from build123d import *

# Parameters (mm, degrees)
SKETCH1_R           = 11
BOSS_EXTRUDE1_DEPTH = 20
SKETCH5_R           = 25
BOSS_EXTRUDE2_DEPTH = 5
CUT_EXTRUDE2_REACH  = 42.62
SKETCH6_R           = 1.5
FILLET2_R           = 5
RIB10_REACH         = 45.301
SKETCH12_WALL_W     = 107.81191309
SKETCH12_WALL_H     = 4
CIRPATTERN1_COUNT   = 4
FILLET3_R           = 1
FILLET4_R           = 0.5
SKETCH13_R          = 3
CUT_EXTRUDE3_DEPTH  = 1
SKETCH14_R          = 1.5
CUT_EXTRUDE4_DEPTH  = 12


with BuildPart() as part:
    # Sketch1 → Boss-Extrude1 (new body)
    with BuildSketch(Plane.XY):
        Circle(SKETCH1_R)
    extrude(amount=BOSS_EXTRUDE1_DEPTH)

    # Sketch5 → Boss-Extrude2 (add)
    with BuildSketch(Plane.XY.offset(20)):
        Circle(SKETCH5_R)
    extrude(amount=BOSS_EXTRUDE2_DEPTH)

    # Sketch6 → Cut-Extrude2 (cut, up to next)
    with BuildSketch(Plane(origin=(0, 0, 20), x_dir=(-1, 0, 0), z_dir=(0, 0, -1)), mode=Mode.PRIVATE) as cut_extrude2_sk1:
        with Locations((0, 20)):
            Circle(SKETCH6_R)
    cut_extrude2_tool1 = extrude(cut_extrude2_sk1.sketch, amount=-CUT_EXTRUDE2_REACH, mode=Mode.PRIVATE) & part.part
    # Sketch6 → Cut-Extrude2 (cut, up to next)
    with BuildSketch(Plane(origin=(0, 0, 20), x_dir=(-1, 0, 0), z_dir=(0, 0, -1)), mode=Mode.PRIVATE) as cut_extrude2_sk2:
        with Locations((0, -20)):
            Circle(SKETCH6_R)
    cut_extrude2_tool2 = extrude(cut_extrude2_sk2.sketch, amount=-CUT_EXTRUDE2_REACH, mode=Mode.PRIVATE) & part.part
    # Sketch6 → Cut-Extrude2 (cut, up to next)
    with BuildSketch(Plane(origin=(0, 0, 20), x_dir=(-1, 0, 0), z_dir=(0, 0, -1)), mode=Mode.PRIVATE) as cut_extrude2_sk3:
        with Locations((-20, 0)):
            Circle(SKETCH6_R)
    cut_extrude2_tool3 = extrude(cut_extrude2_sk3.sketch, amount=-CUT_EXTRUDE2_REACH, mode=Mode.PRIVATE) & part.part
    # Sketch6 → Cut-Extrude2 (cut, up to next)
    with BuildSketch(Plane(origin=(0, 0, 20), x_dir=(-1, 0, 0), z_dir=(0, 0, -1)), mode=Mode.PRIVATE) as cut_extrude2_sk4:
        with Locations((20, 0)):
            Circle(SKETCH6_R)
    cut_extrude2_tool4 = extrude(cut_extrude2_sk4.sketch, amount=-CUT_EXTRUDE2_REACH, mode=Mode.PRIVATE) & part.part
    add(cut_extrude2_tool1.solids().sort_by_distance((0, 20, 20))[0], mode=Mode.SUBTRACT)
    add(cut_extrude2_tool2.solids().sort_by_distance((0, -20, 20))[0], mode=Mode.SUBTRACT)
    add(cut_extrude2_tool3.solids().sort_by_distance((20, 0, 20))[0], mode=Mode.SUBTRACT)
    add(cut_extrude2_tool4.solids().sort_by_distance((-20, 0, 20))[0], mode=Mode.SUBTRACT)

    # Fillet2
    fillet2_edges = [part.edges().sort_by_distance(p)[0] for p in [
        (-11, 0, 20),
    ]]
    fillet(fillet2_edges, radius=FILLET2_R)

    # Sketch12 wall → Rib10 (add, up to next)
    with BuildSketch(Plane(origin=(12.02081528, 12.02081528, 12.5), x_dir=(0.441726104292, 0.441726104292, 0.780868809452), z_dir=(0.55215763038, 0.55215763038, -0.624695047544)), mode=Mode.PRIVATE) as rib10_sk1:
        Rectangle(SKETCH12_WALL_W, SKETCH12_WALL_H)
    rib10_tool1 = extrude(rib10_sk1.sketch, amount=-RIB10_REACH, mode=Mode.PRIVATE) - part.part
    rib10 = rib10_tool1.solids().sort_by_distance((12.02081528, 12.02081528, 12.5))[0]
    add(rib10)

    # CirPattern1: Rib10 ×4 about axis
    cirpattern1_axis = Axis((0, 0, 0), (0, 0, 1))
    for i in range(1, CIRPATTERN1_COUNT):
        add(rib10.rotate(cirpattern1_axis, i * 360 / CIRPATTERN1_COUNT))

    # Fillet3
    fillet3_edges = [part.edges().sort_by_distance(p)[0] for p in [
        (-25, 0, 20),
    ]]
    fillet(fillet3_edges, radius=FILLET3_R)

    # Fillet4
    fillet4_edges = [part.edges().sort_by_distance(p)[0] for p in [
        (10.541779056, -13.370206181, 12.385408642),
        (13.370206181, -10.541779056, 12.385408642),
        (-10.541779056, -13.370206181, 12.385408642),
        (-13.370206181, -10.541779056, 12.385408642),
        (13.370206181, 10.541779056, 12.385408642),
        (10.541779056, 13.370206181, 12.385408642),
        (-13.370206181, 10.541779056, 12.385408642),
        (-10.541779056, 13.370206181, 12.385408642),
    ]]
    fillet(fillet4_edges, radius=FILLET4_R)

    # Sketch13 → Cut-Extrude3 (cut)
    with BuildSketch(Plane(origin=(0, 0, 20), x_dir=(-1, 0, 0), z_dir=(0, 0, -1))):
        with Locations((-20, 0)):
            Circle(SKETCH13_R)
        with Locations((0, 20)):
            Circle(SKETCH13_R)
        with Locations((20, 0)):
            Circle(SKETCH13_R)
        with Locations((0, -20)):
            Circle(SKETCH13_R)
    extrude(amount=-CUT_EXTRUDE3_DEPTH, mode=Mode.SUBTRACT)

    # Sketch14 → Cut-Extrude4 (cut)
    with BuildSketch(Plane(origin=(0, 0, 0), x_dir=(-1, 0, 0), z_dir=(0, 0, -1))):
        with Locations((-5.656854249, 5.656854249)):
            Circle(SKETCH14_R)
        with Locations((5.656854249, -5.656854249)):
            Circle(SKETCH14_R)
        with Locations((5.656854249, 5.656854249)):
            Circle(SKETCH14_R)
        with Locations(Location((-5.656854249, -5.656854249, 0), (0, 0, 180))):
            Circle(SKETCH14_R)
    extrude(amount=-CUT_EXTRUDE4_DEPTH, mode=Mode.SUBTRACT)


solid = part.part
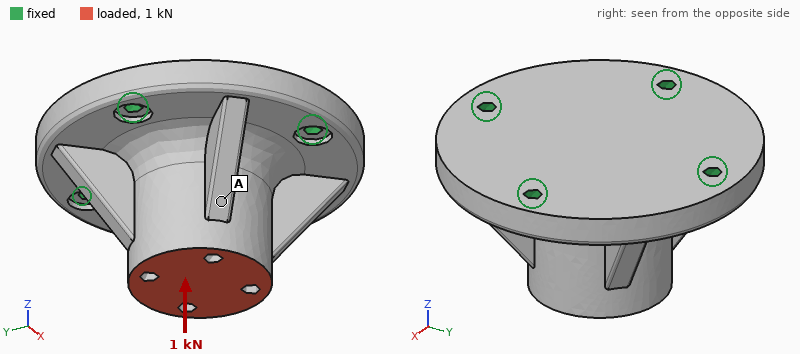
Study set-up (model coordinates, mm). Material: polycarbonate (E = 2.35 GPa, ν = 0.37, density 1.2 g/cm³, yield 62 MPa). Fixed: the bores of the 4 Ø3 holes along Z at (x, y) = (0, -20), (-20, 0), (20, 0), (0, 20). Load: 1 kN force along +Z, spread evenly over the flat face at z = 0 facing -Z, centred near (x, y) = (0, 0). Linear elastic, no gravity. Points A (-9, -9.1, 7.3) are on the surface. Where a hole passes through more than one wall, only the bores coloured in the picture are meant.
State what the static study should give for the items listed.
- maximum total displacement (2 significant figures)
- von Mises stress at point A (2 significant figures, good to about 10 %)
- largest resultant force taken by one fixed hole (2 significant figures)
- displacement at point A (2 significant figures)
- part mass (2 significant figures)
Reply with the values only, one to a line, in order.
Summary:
0.11 mm
3.1 MPa
280 N
0.092 mm
22 g
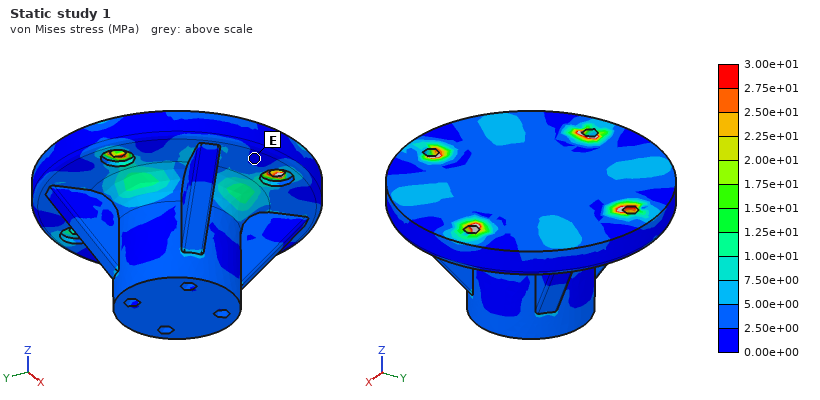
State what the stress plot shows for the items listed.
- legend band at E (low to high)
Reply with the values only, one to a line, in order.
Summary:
0.00e+00 to 2.50e+00 MPa
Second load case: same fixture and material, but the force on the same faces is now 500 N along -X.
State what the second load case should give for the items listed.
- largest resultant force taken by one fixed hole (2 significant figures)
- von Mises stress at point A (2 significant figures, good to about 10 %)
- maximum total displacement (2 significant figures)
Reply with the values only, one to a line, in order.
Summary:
360 N
4.3 MPa
0.22 mm
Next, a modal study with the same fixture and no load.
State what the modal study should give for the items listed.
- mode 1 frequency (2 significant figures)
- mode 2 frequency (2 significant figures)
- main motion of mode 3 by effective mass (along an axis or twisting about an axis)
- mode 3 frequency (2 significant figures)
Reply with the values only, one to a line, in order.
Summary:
3700 Hz
3700 Hz
along Z
4000 Hz
